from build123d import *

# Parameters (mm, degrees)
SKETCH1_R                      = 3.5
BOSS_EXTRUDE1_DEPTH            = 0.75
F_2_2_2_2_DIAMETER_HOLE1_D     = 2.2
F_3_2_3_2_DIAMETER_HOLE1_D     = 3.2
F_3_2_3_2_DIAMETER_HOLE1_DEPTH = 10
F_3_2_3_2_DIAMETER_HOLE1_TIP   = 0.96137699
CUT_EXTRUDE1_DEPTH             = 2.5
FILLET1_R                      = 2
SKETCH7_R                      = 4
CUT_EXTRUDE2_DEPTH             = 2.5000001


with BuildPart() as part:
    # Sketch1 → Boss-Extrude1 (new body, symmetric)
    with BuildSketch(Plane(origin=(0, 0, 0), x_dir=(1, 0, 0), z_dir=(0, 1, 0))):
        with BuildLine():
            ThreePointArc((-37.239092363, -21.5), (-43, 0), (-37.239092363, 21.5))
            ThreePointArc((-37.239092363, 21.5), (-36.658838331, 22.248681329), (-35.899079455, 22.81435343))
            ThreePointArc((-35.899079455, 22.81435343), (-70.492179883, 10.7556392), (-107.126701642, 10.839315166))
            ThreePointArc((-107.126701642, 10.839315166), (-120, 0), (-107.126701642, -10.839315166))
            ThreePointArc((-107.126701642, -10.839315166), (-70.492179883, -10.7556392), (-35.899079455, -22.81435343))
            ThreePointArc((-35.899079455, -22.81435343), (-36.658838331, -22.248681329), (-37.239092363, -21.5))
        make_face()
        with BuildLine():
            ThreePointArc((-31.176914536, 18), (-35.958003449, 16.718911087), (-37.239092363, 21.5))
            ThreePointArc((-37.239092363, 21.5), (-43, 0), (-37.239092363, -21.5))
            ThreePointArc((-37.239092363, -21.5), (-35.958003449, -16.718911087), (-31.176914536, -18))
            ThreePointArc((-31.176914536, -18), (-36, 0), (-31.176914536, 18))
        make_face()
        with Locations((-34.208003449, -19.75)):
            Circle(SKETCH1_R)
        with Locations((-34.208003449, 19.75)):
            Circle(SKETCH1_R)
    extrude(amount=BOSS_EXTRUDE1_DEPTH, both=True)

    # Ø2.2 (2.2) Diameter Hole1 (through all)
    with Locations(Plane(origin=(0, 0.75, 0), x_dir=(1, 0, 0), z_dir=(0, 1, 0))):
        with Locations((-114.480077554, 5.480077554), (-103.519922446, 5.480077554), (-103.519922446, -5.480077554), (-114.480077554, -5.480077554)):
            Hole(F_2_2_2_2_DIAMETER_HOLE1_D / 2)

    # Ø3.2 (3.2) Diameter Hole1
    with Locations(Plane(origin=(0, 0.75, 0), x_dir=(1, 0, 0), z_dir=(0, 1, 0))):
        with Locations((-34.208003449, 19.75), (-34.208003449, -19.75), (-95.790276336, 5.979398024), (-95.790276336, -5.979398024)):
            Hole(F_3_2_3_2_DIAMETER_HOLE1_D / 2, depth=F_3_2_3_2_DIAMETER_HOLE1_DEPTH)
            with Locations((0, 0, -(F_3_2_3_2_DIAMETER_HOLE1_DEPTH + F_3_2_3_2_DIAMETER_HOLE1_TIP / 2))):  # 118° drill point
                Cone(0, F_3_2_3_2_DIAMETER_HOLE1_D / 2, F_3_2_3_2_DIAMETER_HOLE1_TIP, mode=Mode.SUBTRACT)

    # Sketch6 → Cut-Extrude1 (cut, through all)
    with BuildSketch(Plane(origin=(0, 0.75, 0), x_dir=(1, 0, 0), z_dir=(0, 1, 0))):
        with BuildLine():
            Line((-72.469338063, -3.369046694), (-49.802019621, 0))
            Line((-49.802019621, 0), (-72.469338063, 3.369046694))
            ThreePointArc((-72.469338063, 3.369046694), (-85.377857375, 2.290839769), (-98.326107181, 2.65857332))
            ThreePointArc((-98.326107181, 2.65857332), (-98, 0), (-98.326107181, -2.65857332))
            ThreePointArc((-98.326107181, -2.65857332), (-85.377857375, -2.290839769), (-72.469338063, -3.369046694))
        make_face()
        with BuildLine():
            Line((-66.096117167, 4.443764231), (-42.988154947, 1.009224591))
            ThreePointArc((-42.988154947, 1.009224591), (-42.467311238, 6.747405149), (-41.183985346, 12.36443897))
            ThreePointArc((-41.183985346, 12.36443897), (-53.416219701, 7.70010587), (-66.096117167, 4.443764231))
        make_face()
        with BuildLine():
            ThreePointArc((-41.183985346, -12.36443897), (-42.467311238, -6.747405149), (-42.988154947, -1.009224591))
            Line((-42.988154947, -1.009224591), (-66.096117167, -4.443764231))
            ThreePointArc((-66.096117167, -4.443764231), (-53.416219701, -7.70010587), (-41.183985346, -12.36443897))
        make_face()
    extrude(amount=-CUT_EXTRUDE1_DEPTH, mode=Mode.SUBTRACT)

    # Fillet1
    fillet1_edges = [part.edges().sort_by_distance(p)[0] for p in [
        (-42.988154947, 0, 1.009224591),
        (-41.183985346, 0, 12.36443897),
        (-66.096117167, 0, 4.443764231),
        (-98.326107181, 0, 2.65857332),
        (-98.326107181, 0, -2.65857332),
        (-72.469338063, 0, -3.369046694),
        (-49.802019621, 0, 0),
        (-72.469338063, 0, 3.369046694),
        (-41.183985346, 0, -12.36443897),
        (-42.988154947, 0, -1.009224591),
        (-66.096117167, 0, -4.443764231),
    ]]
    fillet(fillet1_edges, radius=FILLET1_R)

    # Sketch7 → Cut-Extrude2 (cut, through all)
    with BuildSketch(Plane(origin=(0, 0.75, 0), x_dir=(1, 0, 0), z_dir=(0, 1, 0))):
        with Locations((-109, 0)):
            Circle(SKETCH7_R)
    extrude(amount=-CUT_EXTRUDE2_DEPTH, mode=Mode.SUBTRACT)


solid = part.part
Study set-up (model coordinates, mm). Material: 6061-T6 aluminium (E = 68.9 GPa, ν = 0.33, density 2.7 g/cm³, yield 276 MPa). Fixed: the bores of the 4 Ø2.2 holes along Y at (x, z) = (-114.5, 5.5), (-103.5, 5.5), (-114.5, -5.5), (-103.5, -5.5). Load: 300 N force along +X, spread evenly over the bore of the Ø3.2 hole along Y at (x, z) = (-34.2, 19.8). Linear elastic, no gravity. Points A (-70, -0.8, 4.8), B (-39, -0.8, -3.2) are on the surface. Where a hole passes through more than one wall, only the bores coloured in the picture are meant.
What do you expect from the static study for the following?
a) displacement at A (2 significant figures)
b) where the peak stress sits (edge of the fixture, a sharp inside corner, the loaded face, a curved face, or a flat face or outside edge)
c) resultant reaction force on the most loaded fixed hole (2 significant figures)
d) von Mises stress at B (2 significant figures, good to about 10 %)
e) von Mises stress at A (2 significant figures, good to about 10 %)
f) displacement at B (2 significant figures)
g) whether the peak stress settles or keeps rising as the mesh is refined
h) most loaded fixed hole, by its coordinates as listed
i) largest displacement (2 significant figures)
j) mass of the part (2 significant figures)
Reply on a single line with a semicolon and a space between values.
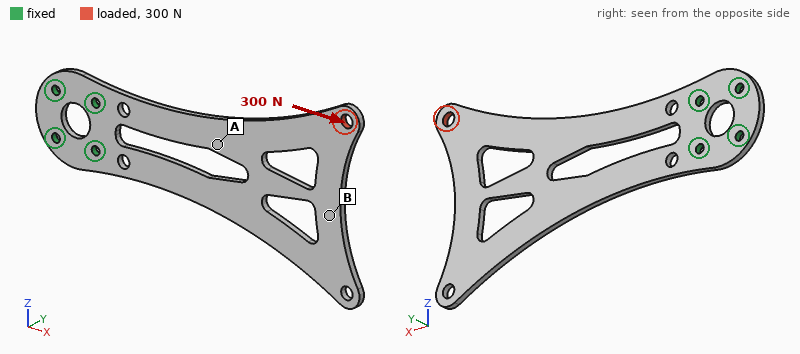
0.096 mm; a sharp inside corner; 510 N; 18 MPa; 44 MPa; 0.27 mm; keeps rising; (-103.5, 5.5); 0.37 mm; 6.7 g
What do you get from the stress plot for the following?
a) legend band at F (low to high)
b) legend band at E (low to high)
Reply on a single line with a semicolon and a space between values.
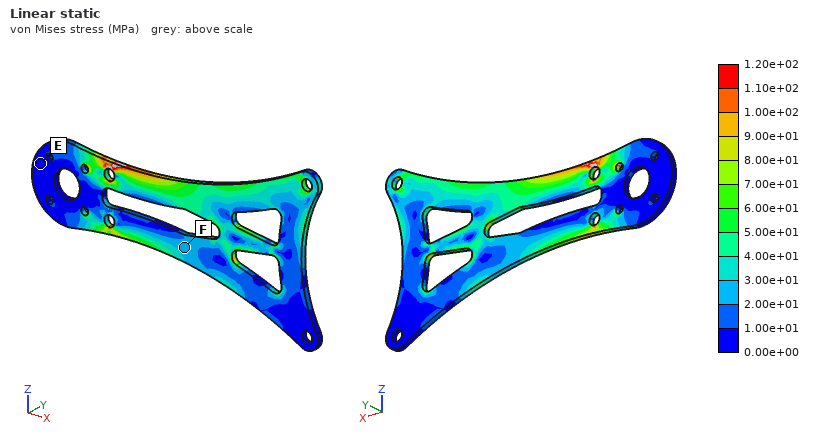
2.00e+01 to 3.00e+01 MPa; 0.00e+00 to 1.00e+01 MPa
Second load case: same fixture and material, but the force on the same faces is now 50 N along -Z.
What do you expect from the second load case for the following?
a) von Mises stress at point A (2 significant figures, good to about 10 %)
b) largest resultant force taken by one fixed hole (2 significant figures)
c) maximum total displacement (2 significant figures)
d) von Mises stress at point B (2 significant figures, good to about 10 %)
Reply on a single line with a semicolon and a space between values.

23 MPa; 200 N; 0.20 mm; 5.8 MPa
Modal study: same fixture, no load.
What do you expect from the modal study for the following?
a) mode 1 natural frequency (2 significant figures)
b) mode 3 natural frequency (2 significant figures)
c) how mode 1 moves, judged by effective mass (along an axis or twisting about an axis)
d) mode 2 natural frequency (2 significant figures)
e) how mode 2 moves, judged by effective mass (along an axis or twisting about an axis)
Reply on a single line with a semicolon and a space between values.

180 Hz; 1400 Hz; along Y; 650 Hz; twisting about X
